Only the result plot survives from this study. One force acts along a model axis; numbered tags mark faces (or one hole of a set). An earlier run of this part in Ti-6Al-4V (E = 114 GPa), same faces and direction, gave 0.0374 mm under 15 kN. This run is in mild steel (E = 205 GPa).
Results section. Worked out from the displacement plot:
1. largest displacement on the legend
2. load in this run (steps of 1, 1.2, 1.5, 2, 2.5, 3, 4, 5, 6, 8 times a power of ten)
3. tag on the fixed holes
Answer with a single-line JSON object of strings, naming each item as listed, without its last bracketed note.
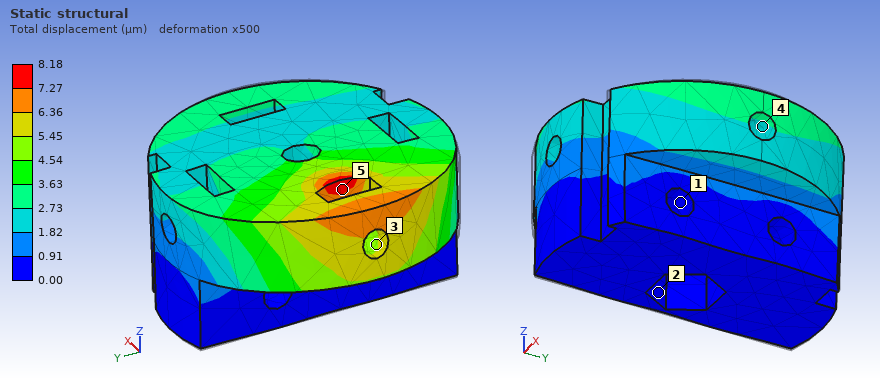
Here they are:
{"largest displacement on the legend": "8.18 µm", "load in this run": "6 kN", "tag on the fixed holes": "1"}
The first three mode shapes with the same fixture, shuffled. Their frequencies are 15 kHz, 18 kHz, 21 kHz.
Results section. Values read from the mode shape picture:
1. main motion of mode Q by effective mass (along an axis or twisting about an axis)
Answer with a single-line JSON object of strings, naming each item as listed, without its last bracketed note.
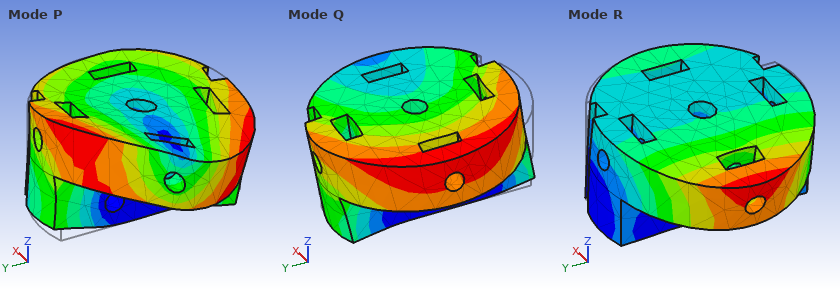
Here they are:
{"main motion of mode Q by effective mass": "along Y"}
